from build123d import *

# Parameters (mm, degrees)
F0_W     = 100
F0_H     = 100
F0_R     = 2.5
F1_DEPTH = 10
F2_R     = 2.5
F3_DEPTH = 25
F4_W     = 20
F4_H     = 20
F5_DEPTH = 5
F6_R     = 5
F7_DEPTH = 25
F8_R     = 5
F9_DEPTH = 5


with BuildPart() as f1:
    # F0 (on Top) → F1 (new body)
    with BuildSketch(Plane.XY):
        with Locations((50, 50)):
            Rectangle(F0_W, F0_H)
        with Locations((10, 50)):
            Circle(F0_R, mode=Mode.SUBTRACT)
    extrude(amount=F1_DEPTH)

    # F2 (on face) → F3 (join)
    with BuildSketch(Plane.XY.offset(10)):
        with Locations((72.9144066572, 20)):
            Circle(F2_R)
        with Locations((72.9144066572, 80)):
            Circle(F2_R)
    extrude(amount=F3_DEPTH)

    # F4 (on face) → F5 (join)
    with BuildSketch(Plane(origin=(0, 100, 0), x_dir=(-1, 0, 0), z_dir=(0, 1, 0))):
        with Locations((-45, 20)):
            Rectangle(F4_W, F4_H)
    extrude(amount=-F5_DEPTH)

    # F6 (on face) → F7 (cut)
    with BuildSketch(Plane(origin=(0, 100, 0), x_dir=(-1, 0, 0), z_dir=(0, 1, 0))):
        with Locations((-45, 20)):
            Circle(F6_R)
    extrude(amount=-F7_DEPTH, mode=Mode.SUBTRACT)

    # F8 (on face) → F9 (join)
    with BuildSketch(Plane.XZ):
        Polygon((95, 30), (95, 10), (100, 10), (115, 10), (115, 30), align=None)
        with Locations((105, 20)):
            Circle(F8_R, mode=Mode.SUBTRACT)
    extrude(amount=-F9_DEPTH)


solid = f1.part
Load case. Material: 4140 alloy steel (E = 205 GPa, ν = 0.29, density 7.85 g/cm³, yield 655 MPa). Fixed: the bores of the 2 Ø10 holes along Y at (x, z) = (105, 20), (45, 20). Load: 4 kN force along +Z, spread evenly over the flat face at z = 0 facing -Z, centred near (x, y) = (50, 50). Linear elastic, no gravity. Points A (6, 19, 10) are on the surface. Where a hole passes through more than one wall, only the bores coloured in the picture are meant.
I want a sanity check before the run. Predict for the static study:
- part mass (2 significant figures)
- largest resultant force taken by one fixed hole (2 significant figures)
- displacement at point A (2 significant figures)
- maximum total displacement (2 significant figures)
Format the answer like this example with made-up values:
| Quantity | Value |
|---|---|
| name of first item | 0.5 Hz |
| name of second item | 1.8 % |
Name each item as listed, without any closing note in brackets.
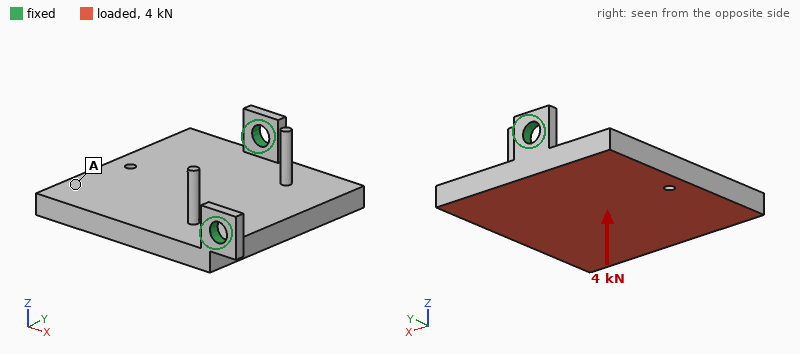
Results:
| Quantity | Value |
|---|---|
| part mass | 820 g |
| largest resultant force taken by one fixed hole | 2.9 kN |
| displacement at point A | 0.40 mm |
| maximum total displacement | 0.49 mm |
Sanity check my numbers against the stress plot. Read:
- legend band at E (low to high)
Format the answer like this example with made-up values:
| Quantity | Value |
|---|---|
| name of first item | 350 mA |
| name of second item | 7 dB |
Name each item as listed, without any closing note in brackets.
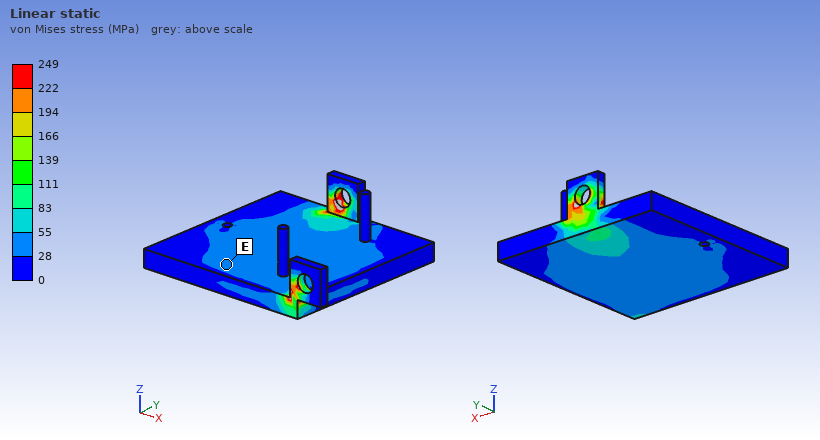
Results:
| Quantity | Value |
|---|---|
| legend band at E | 28 to 55 MPa |
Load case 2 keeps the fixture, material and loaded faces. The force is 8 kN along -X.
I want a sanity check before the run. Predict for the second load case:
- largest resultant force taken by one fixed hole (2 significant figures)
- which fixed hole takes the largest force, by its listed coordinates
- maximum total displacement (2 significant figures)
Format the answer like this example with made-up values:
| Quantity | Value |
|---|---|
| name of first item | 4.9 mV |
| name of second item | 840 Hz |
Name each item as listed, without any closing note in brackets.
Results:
| Quantity | Value |
|---|---|
| largest resultant force taken by one fixed hole | 4.3 kN |
| which fixed hole takes the largest force, by its listed coordinates | (45, 20) |
| maximum total displacement | 0.36 mm |
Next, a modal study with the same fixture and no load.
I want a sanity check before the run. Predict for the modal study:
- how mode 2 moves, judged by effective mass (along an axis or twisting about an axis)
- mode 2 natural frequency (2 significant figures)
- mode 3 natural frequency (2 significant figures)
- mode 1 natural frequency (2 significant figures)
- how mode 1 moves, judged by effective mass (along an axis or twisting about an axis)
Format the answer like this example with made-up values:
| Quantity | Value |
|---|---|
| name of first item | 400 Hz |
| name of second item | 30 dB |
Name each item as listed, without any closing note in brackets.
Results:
| Quantity | Value |
|---|---|
| how mode 2 moves, judged by effective mass | along Z |
| mode 2 natural frequency | 2200 Hz |
| mode 3 natural frequency | 2900 Hz |
| mode 1 natural frequency | 660 Hz |
| how mode 1 moves, judged by effective mass | along Z |
